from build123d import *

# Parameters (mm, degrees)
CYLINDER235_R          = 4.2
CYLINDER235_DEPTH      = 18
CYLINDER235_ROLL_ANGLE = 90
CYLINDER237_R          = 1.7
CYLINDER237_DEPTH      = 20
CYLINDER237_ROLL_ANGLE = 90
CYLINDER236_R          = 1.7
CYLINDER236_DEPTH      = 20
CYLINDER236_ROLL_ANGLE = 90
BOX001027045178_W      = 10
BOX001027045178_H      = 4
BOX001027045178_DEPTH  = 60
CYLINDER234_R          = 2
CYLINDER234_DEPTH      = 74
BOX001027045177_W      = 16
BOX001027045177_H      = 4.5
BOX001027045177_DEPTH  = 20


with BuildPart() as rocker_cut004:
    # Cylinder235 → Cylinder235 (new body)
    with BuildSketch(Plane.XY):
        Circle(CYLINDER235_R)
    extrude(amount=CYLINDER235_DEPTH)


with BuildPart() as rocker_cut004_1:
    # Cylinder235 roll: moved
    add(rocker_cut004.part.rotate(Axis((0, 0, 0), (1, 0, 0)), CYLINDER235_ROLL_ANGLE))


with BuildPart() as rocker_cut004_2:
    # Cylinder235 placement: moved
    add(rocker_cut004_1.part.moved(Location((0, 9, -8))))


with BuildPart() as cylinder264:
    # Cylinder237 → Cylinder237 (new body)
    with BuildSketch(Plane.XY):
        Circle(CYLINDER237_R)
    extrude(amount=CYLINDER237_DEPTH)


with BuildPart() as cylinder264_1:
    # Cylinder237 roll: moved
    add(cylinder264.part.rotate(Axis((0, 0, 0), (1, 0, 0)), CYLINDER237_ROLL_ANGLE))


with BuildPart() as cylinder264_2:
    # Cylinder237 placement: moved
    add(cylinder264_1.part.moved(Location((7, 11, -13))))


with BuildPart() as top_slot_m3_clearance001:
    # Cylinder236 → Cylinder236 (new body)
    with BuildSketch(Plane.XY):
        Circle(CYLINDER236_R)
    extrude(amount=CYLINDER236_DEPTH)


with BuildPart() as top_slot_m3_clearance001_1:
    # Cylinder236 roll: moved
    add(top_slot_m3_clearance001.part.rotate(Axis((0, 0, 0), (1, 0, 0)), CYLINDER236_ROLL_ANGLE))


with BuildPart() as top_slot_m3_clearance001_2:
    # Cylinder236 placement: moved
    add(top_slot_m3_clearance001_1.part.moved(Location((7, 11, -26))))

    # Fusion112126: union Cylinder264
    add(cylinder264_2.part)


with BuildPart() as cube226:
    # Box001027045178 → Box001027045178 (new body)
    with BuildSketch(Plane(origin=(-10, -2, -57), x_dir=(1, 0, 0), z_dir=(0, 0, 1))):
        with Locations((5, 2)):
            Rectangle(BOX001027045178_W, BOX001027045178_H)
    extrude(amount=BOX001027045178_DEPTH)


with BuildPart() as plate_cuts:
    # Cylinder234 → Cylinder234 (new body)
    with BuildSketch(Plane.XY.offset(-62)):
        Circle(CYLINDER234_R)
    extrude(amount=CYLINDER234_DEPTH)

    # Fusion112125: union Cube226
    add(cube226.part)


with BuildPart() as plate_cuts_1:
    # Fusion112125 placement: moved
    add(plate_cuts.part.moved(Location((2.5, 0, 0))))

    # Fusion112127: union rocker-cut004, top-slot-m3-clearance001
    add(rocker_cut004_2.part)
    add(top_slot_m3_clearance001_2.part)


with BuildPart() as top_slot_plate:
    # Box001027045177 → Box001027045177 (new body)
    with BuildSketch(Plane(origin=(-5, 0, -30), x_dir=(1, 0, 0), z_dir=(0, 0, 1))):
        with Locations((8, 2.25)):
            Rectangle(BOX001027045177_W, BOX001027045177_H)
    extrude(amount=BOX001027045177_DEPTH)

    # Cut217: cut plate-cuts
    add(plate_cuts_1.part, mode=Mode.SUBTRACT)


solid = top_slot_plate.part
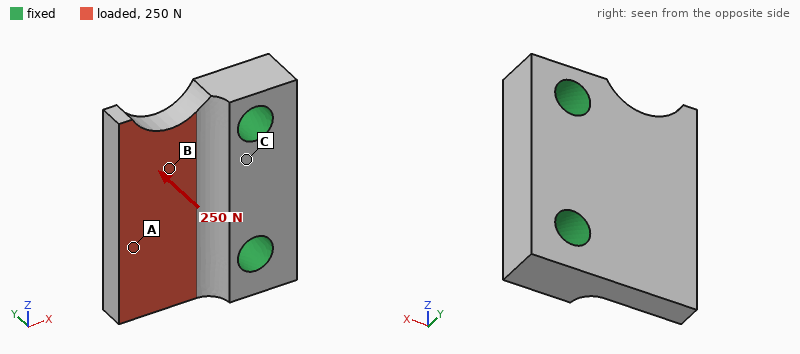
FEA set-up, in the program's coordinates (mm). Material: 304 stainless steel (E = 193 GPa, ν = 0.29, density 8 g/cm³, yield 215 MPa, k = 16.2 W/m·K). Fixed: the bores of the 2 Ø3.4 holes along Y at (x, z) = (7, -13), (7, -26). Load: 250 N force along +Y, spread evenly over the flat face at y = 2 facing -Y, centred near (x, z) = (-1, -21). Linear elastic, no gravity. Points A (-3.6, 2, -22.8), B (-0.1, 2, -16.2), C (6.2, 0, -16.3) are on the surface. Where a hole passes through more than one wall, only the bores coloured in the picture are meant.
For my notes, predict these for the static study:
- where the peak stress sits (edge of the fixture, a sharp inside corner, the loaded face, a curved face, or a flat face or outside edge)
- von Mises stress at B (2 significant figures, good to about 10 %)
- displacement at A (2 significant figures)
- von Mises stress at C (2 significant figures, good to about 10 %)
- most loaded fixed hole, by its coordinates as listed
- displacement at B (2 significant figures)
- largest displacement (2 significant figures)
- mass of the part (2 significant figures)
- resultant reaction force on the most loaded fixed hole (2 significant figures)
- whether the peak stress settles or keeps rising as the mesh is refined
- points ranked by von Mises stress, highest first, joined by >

edge of the fixture
23 MPa
7.3 µm
15 MPa
(7, -26)
3.6 µm
9.0 µm
7.7 g
140 N
keeps rising
B > C > A
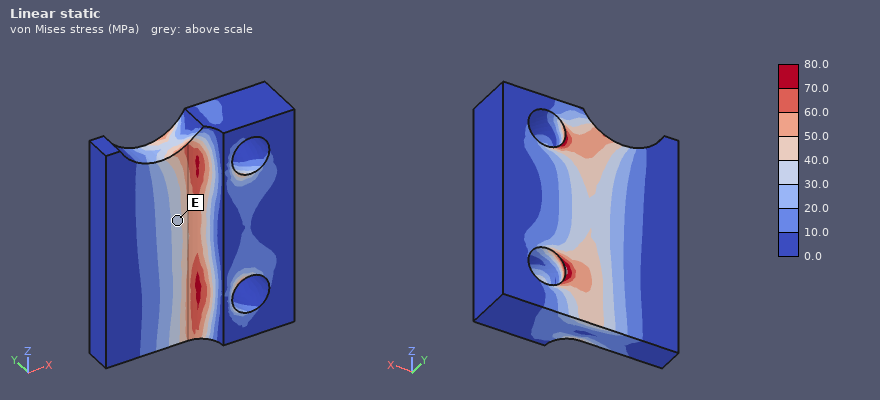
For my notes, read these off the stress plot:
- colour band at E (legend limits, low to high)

30.0 to 40.0 MPa
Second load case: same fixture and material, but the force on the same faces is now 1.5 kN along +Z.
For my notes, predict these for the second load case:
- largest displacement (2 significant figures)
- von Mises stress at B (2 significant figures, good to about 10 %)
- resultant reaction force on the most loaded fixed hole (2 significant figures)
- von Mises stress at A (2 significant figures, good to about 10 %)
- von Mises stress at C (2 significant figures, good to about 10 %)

13 µm
90 MPa
1.1 kN
49 MPa
21 MPa
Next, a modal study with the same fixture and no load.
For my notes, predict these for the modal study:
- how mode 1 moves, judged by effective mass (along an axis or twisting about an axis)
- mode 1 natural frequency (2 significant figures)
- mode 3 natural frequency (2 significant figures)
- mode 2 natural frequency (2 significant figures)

along Y
19 kHz
51 kHz
29 kHz
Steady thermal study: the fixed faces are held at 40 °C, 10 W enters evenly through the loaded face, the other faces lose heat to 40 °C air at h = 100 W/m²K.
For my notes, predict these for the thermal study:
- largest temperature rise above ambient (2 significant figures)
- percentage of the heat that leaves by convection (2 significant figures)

83 K
19 %
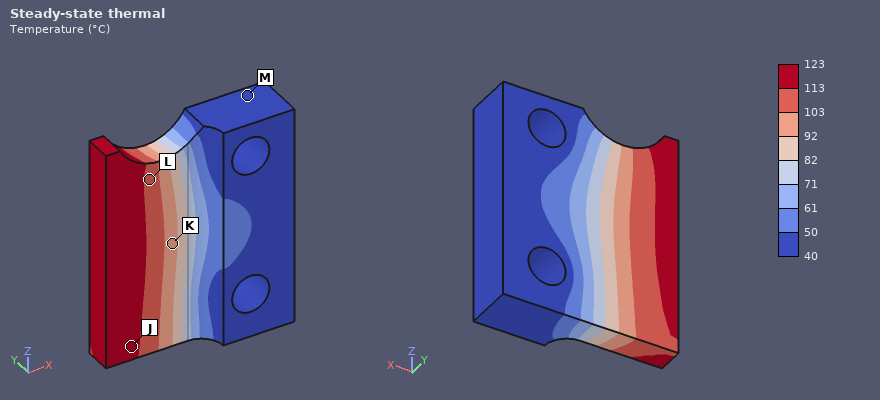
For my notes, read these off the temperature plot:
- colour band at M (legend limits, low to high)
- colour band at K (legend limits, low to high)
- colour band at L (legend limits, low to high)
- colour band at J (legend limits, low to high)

40 to 50 °C
92 to 103 °C
103 to 113 °C
113 to 123 °C
